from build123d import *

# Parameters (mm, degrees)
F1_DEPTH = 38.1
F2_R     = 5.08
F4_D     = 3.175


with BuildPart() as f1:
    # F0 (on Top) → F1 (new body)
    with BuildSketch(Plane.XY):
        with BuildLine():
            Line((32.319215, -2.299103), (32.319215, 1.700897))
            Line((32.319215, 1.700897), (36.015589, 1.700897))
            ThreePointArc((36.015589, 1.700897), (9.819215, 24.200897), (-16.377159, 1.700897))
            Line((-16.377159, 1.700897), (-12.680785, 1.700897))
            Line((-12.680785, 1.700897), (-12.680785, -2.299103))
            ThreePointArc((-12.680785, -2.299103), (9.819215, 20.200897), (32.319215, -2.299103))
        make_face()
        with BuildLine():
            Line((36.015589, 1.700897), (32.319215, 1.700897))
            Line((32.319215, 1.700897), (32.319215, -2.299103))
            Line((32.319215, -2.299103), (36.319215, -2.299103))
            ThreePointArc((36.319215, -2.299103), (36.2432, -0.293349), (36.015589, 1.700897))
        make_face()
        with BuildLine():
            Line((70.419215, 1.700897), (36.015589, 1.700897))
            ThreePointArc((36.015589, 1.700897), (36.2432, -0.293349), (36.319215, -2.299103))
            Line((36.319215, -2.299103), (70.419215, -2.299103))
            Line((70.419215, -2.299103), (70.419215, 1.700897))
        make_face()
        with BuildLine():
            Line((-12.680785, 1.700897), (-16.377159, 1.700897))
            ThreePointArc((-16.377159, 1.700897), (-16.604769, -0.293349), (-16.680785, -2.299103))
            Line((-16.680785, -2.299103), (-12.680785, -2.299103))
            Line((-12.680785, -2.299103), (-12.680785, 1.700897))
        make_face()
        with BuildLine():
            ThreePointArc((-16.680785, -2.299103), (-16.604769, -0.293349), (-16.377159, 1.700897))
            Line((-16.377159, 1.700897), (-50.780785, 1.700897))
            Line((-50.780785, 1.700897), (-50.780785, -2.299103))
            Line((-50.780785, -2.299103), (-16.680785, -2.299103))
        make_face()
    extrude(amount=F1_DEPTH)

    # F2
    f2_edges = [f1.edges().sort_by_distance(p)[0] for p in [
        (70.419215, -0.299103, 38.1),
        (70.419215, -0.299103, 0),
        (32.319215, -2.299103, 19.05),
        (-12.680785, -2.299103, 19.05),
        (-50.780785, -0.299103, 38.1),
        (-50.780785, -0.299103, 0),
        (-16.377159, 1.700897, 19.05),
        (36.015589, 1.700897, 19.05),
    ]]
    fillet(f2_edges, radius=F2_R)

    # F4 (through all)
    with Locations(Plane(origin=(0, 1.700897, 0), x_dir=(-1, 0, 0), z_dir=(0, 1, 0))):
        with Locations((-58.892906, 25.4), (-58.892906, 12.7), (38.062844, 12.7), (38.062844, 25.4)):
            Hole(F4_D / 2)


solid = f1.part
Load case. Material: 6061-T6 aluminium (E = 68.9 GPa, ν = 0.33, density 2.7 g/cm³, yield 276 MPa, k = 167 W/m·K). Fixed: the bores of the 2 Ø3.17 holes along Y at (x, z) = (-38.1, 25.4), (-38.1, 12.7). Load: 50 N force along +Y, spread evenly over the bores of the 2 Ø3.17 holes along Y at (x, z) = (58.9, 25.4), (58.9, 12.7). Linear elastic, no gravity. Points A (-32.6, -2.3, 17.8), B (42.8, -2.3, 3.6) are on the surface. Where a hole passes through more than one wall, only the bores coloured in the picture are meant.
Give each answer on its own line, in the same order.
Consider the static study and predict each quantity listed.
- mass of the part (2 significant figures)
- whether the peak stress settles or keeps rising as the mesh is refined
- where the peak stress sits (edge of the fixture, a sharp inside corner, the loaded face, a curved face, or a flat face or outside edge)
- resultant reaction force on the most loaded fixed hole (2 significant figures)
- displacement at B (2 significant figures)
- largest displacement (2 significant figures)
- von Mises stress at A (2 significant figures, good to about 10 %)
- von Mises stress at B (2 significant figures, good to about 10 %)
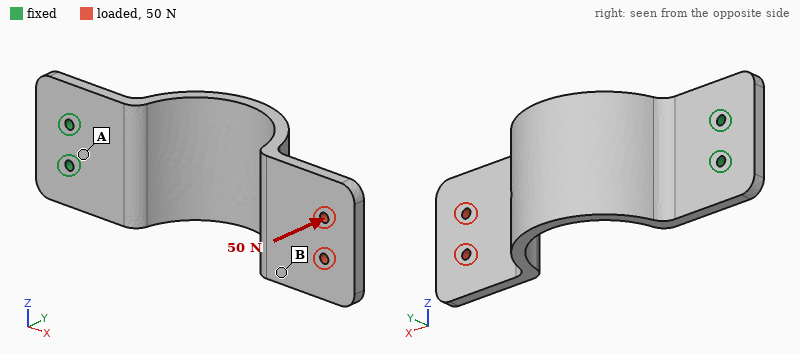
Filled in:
59 g
keeps rising
edge of the fixture
30 N
0.93 mm
1.4 mm
43 MPa
7.7 MPa
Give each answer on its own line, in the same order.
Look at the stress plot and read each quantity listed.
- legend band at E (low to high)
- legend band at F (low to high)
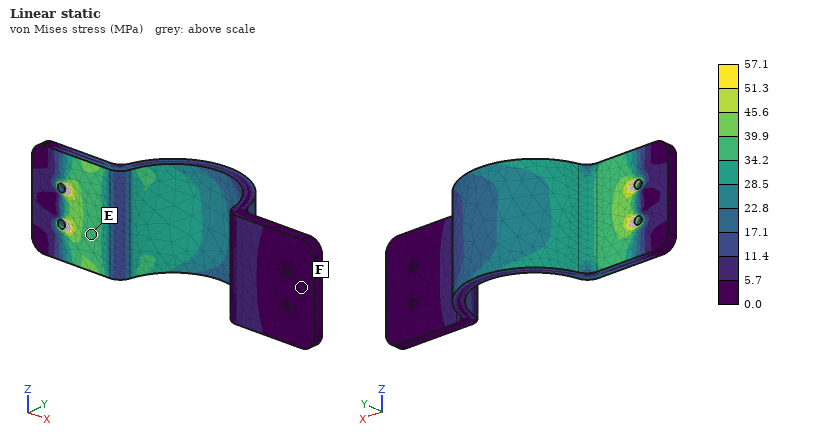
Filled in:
34.2 to 39.9 MPa
0.0 to 5.7 MPa
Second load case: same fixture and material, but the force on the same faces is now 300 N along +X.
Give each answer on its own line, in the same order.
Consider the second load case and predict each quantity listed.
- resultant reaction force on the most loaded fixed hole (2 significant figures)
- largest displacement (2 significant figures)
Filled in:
150 N
1.3 mm
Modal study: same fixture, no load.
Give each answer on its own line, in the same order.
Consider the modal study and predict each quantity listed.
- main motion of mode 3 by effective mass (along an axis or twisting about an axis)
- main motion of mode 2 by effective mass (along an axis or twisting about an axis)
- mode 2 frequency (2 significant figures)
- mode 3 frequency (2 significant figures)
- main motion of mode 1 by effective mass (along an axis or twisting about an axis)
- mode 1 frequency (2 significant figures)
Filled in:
along X
along Z
570 Hz
950 Hz
along Y
250 Hz
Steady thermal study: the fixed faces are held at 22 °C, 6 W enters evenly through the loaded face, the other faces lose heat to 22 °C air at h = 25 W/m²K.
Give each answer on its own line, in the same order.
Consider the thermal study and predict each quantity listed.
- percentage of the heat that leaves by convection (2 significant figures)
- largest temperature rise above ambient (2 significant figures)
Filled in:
44 %
20 K
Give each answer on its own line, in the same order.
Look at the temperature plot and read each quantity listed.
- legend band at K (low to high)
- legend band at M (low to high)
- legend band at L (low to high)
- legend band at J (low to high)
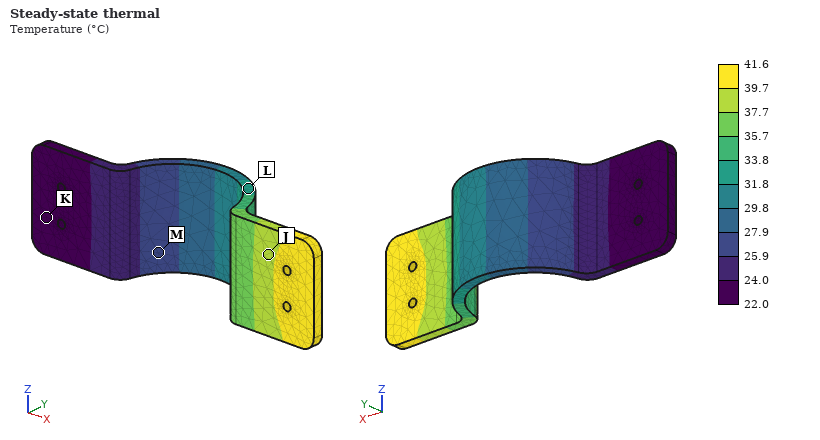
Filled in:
22.0 to 24.0 °C
25.9 to 27.9 °C
31.8 to 33.8 °C
37.7 to 39.7 °C
